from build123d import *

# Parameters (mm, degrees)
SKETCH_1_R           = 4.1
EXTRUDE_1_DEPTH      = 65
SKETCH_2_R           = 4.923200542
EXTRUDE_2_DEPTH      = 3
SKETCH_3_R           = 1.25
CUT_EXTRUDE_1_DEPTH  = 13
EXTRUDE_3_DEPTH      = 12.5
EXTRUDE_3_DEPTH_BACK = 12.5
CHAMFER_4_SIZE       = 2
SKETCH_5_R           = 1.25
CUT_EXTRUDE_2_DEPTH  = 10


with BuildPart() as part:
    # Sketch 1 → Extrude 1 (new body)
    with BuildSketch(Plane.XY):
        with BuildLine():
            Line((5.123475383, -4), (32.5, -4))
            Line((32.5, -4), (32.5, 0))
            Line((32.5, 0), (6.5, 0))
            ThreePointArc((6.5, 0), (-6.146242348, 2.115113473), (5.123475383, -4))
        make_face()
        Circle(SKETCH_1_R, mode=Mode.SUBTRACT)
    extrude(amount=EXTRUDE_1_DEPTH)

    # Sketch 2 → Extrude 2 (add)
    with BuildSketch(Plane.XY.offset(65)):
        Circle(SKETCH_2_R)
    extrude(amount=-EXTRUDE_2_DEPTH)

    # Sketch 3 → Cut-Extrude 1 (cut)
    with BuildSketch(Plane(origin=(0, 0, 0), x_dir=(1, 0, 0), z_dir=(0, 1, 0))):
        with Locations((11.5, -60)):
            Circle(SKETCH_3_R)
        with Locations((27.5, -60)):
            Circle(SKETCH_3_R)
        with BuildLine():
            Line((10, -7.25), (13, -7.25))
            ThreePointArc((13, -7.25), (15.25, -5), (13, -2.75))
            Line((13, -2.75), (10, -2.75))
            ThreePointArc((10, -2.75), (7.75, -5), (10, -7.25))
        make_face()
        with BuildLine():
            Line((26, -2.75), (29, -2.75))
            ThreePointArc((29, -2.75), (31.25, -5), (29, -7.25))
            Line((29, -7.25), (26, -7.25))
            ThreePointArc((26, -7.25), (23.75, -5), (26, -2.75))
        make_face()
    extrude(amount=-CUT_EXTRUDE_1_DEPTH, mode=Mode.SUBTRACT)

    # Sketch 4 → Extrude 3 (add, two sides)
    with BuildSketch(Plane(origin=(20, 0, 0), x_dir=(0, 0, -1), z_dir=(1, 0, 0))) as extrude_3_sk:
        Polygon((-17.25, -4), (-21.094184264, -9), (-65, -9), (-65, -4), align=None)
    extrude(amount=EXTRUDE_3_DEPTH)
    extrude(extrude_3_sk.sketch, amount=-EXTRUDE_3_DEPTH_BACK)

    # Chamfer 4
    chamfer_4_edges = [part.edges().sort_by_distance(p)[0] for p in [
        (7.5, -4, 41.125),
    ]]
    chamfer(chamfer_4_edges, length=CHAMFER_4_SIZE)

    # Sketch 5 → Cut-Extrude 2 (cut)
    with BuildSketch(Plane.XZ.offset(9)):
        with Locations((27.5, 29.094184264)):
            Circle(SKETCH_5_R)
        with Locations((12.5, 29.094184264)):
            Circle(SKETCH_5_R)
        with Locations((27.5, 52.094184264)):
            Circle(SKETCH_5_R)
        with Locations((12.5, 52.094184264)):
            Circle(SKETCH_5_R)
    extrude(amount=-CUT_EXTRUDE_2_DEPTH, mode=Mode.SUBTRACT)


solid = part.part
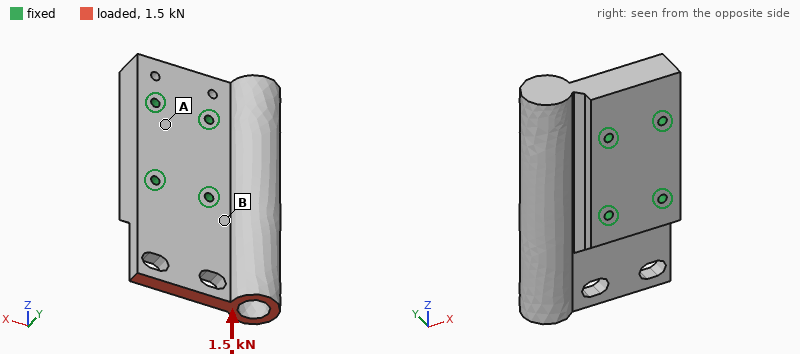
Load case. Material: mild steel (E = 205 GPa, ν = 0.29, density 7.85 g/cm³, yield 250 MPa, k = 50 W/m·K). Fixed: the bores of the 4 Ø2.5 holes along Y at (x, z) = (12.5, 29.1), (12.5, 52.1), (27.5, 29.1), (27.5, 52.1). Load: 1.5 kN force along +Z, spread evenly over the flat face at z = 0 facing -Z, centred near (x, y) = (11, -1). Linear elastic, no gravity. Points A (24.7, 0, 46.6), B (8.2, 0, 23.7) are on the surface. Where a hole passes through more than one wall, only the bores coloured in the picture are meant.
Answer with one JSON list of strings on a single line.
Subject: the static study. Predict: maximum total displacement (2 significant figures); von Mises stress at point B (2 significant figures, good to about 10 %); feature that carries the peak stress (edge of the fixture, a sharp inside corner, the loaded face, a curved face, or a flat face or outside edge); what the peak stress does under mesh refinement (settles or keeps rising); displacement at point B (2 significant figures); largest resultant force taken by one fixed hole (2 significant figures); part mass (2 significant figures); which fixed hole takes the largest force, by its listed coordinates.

["3.2 µm", "11 MPa", "a sharp inside corner", "keeps rising", "0.73 µm", "870 N", "140 g", "(12.5, 29.1)"]
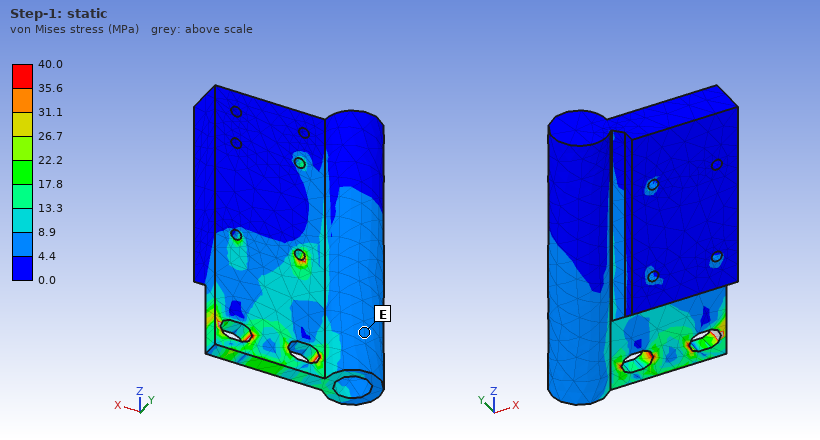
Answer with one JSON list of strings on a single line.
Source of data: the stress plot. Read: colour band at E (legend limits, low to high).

["4.4 to 8.9 MPa"]
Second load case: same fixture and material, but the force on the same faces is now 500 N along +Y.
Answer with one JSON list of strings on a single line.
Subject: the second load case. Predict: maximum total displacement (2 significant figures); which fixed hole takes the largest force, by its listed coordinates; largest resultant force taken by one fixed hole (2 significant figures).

["26 µm", "(12.5, 29.1)", "760 N"]
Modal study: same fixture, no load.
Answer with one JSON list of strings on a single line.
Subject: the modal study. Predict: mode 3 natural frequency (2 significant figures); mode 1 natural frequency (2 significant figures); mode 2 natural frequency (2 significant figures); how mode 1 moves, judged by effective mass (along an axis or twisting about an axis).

["12 kHz", "7200 Hz", "9200 Hz", "along Y"]
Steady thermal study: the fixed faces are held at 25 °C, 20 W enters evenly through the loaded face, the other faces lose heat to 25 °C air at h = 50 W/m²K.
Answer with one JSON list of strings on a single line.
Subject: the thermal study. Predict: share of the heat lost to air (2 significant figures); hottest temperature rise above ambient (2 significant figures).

["27 %", "67 K"]
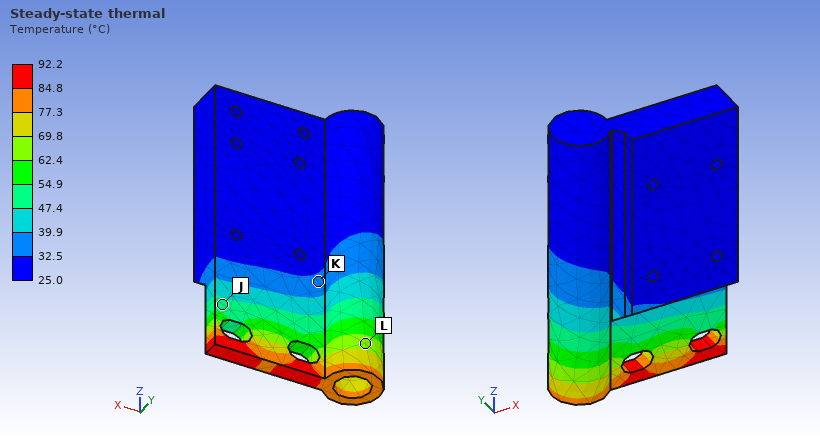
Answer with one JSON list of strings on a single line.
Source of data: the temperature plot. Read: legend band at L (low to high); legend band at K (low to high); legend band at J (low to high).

["62.4 to 69.8 °C", "32.5 to 39.9 °C", "47.4 to 54.9 °C"]
